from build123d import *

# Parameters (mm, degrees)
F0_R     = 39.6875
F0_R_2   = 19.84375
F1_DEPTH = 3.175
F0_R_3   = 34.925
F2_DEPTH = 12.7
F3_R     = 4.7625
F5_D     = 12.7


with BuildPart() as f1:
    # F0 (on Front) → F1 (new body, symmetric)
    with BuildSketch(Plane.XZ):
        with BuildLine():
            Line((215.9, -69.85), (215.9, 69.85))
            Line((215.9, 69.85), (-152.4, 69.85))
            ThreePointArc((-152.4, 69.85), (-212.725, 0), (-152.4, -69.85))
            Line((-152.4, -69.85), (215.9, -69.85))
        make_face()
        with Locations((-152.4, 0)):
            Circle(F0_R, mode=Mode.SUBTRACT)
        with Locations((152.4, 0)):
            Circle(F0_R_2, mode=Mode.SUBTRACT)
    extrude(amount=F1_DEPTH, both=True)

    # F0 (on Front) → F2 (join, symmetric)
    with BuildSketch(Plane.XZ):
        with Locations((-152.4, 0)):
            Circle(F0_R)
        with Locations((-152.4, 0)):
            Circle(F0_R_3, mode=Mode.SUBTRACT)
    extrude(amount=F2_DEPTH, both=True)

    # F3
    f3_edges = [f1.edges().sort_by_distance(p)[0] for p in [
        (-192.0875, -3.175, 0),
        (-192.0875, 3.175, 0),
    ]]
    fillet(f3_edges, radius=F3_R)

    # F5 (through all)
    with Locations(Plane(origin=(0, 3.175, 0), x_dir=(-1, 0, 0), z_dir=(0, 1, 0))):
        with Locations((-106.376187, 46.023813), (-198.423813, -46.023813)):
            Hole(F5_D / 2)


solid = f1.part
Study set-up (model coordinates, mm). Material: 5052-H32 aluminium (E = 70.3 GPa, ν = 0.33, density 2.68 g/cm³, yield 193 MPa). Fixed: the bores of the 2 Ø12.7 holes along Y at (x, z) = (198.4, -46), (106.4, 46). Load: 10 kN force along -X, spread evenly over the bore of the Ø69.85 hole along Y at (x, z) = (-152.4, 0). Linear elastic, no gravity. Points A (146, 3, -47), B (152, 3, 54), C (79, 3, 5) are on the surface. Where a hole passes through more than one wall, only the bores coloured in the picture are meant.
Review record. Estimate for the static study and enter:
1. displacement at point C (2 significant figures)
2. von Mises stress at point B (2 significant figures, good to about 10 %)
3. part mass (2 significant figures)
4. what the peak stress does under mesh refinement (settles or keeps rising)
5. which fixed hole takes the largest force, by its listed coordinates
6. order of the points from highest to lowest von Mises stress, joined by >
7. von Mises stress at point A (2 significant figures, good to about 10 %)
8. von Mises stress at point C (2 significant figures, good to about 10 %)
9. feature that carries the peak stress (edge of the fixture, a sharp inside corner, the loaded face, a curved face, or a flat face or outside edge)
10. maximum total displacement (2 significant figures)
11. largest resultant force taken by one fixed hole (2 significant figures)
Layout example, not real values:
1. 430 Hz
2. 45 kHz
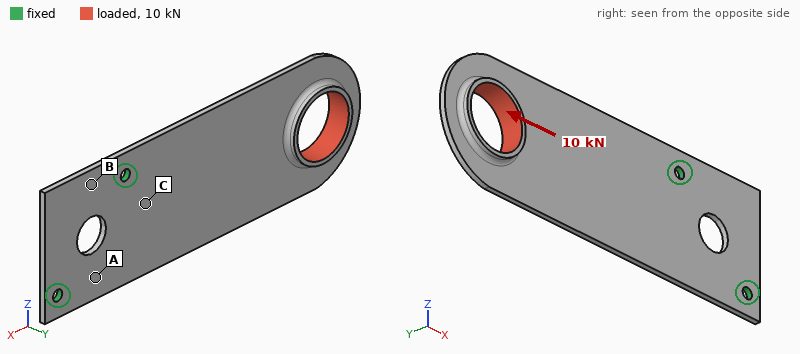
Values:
1. 18 µm
2. 3.3 MPa
3. 960 g
4. keeps rising
5. (106.4, 46)
6. A > C > B
7. 14 MPa
8. 8.5 MPa
9. edge of the fixture
10. 95 µm
11. 5.6 kN
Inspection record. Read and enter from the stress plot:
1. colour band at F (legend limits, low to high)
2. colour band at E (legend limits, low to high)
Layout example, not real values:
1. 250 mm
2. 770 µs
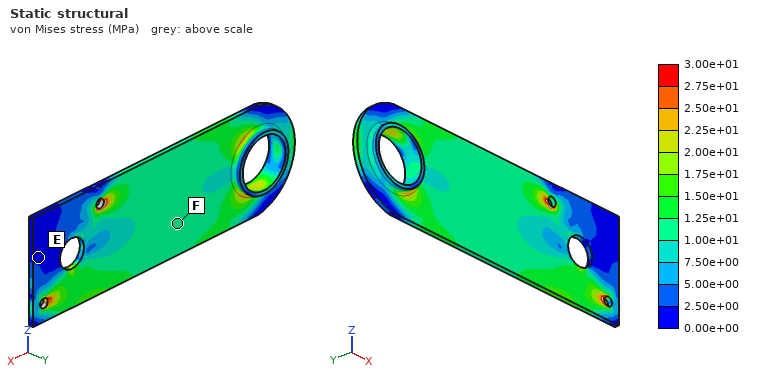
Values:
1. 1.00e+01 to 1.25e+01 MPa
2. 0.00e+00 to 2.50e+00 MPa
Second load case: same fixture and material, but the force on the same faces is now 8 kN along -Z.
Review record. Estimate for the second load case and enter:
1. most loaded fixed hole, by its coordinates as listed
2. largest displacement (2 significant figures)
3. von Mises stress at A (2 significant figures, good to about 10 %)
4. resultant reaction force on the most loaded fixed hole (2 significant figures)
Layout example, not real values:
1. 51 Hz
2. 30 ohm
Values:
1. (106.4, 46)
2. 1.1 mm
3. 62 MPa
4. 21 kN
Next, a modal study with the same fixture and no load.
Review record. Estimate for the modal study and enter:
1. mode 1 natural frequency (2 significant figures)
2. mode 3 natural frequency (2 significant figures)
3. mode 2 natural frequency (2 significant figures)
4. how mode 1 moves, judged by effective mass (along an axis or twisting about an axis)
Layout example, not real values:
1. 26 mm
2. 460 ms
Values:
1. 52 Hz
2. 320 Hz
3. 220 Hz
4. along Y
